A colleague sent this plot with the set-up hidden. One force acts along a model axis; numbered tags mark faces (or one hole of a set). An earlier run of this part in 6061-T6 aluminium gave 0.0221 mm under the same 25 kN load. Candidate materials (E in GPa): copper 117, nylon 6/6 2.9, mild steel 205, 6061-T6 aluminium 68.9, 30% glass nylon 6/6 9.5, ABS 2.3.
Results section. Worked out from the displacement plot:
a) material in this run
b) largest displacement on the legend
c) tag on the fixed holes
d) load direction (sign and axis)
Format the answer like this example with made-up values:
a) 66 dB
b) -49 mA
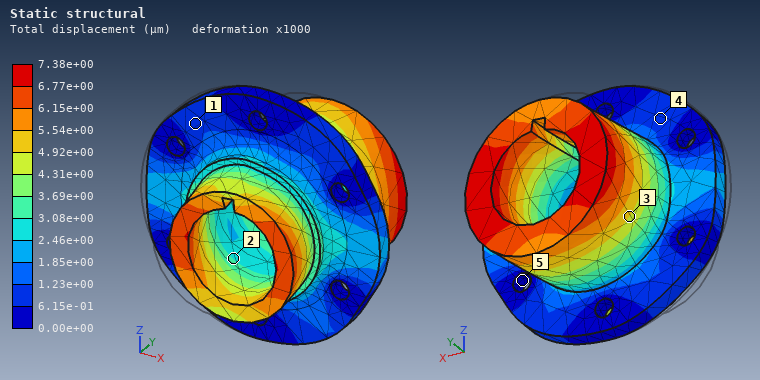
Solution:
a) mild steel
b) 7.38e+00 µm
c) 5
d) +X
